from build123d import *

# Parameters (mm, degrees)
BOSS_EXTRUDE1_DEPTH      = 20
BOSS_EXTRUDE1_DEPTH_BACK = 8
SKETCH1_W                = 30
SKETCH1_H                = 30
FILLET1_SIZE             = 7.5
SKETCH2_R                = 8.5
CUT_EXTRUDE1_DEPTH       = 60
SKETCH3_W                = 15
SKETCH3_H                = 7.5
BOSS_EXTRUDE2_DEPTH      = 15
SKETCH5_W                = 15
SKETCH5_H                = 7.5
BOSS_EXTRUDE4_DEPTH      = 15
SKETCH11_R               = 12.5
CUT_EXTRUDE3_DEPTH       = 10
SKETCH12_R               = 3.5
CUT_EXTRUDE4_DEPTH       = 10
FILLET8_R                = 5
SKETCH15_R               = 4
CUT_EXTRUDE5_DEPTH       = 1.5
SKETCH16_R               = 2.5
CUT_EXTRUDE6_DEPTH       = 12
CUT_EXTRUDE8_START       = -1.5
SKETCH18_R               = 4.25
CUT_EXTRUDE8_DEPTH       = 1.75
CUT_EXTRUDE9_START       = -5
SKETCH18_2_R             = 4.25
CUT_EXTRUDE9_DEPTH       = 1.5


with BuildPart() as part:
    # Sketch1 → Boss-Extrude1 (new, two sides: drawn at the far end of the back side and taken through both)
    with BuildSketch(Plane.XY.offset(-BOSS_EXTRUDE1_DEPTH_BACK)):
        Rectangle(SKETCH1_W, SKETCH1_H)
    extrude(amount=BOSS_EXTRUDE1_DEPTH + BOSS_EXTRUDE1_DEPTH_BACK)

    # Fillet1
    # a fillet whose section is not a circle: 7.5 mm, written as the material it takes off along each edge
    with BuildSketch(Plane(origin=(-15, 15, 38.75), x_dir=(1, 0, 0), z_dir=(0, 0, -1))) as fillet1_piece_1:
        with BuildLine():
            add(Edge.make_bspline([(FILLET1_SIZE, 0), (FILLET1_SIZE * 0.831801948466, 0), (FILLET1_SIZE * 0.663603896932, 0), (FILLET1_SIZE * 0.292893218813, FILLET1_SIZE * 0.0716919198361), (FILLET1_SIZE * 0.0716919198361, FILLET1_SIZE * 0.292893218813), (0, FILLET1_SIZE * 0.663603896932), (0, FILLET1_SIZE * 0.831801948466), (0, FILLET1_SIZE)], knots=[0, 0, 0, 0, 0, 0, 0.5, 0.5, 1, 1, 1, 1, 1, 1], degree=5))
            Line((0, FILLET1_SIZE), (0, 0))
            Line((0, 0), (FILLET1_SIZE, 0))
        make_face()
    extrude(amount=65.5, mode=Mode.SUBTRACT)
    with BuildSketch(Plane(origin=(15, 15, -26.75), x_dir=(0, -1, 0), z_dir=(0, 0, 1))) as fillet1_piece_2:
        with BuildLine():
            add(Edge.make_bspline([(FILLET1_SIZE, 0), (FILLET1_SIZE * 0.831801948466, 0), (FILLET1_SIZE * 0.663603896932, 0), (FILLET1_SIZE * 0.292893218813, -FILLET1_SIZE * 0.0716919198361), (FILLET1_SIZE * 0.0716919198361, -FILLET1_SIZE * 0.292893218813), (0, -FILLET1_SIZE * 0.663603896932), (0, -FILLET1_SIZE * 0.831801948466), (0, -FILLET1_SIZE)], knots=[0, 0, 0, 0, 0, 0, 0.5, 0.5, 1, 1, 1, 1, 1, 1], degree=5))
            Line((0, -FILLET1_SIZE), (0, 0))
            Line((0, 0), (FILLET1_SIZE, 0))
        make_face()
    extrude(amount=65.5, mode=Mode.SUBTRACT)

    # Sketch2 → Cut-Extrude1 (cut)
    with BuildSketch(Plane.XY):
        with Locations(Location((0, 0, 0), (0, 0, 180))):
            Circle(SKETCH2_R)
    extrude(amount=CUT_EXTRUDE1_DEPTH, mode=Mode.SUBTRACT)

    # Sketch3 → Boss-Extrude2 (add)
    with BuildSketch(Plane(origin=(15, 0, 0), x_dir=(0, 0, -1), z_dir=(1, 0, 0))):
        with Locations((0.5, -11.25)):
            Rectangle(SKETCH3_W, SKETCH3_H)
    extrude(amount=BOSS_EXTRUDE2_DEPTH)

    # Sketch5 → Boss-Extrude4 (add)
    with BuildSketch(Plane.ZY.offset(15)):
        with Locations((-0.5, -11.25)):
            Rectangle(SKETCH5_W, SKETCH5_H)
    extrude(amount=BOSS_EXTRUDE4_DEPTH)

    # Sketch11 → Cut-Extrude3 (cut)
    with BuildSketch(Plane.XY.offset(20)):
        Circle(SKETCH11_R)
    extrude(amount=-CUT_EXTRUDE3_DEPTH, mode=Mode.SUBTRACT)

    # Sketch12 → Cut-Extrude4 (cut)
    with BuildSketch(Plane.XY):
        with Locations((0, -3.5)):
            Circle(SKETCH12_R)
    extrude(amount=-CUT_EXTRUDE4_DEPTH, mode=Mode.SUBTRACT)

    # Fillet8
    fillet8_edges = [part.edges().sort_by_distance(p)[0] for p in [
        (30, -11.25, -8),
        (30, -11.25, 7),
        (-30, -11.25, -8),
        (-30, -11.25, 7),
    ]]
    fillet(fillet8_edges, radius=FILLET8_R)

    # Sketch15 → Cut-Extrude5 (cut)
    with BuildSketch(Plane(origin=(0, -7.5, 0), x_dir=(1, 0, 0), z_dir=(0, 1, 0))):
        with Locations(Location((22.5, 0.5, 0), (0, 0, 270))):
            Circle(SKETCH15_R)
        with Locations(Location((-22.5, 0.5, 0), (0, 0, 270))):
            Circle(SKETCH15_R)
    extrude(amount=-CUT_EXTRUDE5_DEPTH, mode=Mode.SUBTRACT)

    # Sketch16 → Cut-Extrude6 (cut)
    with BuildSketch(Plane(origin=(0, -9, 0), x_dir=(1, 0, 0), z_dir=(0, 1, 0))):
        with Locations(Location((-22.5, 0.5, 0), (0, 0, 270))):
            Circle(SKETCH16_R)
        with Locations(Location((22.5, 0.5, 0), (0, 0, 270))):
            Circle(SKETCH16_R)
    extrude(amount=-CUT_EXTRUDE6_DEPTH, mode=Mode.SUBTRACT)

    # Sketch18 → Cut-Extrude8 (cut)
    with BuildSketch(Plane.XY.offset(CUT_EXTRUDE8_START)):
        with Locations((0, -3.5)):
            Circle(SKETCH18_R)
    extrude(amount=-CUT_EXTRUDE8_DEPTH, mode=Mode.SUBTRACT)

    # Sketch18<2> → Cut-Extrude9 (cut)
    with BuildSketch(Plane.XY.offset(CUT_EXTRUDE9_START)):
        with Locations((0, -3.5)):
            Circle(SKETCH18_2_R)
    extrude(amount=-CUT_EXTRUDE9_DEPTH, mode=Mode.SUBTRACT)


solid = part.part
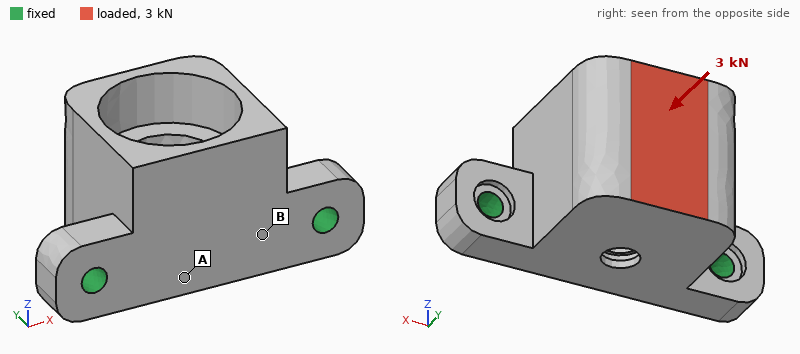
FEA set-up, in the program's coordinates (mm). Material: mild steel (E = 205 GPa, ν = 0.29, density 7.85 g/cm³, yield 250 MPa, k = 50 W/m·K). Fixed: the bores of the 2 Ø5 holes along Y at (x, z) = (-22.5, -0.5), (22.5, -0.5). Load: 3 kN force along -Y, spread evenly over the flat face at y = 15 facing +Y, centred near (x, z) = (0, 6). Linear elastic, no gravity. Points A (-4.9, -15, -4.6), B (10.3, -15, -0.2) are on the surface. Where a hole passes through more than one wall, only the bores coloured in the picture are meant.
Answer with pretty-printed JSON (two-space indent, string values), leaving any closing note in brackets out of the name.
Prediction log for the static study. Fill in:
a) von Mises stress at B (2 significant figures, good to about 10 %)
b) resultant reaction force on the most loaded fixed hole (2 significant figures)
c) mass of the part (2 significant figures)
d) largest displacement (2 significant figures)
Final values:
{
  "von Mises stress at B": "24 MPa",
  "resultant reaction force on the most loaded fixed hole": "1.6 kN",
  "mass of the part": "160 g",
  "largest displacement": "37 µm"
}
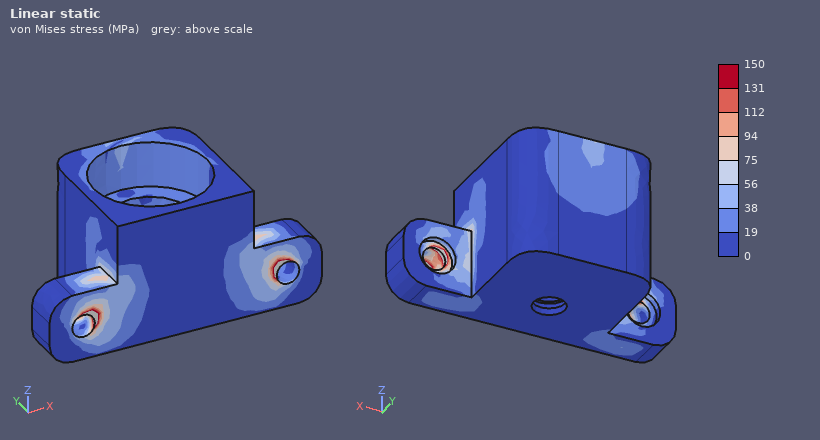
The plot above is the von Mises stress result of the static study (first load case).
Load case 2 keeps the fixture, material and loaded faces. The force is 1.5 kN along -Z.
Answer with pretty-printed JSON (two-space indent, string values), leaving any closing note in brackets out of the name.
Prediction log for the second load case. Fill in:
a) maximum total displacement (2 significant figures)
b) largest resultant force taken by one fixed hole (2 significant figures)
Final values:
{
  "maximum total displacement": "63 µm",
  "largest resultant force taken by one fixed hole": "770 N"
}
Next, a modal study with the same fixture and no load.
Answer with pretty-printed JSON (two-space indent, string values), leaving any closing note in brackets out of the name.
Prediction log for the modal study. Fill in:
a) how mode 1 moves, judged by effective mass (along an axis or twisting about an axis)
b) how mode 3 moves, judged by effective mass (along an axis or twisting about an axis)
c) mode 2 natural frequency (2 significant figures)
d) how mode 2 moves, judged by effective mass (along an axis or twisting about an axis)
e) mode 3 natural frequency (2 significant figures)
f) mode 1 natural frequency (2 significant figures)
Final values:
{
  "how mode 1 moves, judged by effective mass": "along Z",
  "how mode 3 moves, judged by effective mass": "along Y",
  "mode 2 natural frequency": "11 kHz",
  "how mode 2 moves, judged by effective mass": "along X",
  "mode 3 natural frequency": "12 kHz",
  "mode 1 natural frequency": "3700 Hz"
}
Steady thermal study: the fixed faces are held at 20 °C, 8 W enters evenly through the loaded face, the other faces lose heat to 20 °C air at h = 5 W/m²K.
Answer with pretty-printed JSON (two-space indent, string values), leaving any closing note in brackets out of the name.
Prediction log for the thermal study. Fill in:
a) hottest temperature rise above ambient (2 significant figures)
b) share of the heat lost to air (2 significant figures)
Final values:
{
  "hottest temperature rise above ambient": "20 K",
  "share of the heat lost to air": "4.1 %"
}
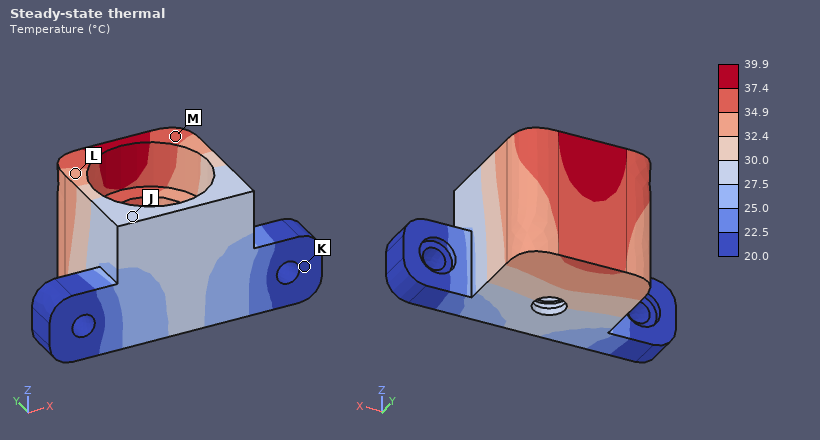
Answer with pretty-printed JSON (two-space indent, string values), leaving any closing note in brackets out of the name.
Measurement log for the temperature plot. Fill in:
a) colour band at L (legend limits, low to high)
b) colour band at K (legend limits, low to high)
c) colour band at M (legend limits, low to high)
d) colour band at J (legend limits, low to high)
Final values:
{
  "colour band at L": "32.4 to 34.9 °C",
  "colour band at K": "20.0 to 22.5 °C",
  "colour band at M": "34.9 to 37.4 °C",
  "colour band at J": "27.5 to 30.0 °C"
}
